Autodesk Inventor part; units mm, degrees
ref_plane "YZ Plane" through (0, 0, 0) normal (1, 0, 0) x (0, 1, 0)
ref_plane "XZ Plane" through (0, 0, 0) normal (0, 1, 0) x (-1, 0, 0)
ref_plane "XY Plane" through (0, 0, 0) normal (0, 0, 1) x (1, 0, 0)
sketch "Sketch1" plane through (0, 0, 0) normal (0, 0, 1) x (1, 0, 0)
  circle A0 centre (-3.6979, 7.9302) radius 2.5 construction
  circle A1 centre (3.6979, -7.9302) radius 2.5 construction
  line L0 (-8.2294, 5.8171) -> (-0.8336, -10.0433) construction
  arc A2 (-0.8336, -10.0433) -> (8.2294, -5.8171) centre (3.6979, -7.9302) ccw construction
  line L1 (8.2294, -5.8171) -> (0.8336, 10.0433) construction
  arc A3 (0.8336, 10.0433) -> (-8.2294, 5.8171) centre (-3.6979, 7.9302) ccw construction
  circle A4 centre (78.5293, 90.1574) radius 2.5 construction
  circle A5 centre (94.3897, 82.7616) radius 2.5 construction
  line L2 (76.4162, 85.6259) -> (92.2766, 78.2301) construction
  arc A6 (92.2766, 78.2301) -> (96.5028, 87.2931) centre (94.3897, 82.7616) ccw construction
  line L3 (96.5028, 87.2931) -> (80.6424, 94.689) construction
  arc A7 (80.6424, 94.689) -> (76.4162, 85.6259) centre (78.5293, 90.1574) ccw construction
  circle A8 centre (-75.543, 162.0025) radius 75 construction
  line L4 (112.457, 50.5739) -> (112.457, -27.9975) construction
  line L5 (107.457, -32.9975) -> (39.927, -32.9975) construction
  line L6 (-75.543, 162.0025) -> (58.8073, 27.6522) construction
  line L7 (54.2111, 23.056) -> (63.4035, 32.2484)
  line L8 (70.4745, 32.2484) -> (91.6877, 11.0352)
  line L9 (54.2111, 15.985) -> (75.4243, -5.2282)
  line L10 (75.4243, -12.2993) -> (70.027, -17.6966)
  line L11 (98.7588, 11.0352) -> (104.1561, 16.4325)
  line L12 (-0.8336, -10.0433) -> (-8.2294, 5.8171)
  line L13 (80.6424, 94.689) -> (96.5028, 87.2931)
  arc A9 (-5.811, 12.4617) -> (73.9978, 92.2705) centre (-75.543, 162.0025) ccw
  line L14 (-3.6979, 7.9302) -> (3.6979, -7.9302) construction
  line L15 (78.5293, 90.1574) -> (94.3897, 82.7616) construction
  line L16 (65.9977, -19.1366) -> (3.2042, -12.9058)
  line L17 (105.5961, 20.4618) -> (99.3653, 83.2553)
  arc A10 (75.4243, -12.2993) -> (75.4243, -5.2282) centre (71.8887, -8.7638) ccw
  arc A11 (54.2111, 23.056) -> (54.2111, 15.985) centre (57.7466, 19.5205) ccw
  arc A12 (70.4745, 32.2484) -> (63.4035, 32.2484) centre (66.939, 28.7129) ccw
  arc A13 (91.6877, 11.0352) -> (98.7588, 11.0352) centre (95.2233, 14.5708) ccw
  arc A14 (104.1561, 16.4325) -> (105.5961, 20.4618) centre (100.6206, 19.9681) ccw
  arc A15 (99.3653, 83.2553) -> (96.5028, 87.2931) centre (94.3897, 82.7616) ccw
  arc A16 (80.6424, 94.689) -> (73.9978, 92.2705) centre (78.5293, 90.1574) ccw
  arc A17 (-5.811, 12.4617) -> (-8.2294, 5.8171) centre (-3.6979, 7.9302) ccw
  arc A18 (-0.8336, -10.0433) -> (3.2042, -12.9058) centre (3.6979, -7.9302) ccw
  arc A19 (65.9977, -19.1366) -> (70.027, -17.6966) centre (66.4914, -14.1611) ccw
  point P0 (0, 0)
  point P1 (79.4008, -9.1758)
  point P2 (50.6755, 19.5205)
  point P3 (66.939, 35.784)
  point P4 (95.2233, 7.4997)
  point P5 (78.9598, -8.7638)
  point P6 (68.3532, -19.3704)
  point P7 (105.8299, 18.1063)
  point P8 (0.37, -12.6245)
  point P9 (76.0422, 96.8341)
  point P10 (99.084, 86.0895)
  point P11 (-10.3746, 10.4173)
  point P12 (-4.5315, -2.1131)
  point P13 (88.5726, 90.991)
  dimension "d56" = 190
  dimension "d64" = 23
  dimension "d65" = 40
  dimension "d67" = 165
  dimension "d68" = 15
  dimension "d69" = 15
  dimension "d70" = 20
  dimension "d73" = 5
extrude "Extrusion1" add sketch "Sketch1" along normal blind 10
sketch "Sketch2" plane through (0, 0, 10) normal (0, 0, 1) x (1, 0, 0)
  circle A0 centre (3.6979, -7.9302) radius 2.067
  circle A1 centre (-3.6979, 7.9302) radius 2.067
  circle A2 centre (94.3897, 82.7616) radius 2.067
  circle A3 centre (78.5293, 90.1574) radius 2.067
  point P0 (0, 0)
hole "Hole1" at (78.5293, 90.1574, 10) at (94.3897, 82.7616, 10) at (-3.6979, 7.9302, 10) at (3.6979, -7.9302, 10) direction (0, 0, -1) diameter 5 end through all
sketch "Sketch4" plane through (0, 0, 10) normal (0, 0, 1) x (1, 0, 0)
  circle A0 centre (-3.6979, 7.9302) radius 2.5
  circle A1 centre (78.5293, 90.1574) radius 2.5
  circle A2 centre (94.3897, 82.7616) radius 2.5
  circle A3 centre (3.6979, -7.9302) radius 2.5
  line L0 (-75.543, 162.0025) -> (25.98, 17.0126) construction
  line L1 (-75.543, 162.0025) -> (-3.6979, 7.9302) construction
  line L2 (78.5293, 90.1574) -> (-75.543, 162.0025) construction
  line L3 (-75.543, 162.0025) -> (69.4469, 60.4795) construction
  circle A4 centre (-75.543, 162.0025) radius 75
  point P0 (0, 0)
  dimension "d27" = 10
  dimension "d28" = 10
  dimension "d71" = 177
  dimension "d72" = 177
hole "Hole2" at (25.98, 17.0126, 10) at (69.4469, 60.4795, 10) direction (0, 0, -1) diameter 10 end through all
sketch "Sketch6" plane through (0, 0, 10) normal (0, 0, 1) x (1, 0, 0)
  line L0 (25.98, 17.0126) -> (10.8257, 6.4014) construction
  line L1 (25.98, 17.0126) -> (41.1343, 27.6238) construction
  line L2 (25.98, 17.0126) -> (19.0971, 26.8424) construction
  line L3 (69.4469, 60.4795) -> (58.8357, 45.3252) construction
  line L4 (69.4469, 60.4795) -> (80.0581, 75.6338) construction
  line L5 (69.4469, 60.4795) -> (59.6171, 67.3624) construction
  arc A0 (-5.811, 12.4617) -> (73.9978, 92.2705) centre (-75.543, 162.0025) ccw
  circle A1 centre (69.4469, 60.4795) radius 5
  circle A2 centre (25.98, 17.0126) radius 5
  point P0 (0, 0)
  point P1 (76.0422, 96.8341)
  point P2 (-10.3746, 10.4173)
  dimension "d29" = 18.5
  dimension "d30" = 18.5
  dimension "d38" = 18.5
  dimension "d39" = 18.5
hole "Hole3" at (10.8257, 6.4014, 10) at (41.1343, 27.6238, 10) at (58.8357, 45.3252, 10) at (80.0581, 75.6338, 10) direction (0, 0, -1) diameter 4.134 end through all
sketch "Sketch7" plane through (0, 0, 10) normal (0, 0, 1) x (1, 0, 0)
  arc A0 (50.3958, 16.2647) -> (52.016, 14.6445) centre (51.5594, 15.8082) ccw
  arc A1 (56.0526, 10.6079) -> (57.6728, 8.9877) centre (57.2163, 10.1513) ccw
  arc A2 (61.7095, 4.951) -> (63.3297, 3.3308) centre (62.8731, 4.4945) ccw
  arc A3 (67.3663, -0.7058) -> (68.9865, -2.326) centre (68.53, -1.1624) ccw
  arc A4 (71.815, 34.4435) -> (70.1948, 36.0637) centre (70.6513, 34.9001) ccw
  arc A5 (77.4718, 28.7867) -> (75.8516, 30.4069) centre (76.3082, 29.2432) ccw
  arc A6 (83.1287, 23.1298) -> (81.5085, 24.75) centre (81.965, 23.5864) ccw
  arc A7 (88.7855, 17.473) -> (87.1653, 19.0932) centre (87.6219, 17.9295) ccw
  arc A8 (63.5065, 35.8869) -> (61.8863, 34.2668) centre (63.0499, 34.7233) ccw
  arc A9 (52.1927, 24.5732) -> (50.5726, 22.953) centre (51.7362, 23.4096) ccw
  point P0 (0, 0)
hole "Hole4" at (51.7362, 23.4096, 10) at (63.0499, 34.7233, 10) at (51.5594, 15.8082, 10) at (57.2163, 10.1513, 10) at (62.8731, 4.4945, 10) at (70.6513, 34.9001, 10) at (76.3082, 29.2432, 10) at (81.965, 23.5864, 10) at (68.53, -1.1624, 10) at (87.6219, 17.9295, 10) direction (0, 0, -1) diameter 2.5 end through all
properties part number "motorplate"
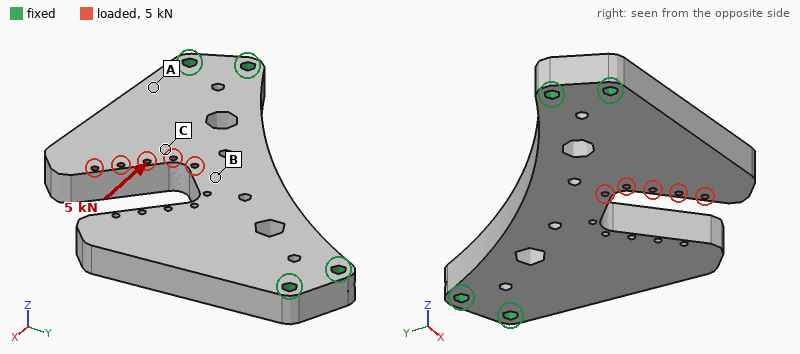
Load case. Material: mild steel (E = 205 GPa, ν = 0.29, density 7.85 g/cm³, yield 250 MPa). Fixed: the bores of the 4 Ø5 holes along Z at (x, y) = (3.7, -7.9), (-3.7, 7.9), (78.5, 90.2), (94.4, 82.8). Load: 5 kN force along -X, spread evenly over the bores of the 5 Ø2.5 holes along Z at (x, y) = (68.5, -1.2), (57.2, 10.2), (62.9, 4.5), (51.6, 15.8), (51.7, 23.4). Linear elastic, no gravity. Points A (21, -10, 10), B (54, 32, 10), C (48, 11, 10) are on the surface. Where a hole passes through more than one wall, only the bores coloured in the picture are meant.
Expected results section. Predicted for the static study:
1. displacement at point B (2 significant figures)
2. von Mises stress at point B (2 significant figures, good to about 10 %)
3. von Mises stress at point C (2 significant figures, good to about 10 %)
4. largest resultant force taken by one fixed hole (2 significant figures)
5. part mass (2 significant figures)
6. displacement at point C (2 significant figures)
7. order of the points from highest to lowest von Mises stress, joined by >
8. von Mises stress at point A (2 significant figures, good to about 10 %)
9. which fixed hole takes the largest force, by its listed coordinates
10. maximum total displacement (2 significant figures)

6.6 µm
4.6 MPa
14 MPa
3.1 kN
470 g
7.1 µm
C > A > B
8.8 MPa
(-3.7, 7.9)
11 µm
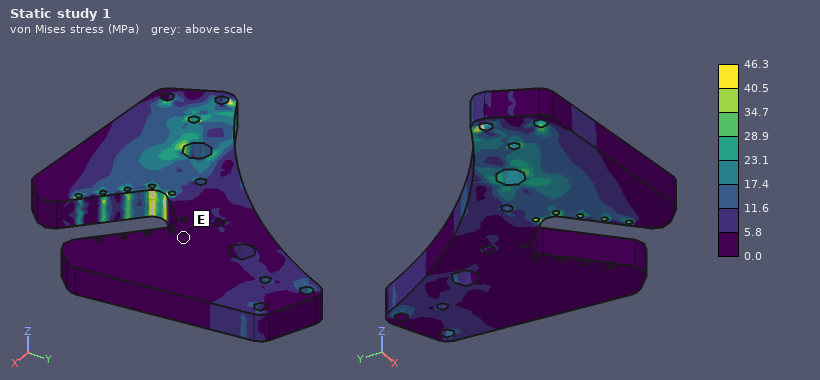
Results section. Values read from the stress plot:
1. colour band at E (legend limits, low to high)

0.0 to 5.8 MPa
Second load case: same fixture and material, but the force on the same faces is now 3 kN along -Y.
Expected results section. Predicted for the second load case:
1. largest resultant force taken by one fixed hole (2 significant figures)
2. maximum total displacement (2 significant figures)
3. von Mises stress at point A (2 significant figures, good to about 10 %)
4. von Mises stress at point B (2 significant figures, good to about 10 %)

2.8 kN
23 µm
13 MPa
22 MPa
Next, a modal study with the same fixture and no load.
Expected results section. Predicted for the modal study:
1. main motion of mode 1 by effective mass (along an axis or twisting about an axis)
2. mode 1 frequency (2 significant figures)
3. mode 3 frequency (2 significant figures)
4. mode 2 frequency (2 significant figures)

along Z
1800 Hz
4300 Hz
2900 Hz
